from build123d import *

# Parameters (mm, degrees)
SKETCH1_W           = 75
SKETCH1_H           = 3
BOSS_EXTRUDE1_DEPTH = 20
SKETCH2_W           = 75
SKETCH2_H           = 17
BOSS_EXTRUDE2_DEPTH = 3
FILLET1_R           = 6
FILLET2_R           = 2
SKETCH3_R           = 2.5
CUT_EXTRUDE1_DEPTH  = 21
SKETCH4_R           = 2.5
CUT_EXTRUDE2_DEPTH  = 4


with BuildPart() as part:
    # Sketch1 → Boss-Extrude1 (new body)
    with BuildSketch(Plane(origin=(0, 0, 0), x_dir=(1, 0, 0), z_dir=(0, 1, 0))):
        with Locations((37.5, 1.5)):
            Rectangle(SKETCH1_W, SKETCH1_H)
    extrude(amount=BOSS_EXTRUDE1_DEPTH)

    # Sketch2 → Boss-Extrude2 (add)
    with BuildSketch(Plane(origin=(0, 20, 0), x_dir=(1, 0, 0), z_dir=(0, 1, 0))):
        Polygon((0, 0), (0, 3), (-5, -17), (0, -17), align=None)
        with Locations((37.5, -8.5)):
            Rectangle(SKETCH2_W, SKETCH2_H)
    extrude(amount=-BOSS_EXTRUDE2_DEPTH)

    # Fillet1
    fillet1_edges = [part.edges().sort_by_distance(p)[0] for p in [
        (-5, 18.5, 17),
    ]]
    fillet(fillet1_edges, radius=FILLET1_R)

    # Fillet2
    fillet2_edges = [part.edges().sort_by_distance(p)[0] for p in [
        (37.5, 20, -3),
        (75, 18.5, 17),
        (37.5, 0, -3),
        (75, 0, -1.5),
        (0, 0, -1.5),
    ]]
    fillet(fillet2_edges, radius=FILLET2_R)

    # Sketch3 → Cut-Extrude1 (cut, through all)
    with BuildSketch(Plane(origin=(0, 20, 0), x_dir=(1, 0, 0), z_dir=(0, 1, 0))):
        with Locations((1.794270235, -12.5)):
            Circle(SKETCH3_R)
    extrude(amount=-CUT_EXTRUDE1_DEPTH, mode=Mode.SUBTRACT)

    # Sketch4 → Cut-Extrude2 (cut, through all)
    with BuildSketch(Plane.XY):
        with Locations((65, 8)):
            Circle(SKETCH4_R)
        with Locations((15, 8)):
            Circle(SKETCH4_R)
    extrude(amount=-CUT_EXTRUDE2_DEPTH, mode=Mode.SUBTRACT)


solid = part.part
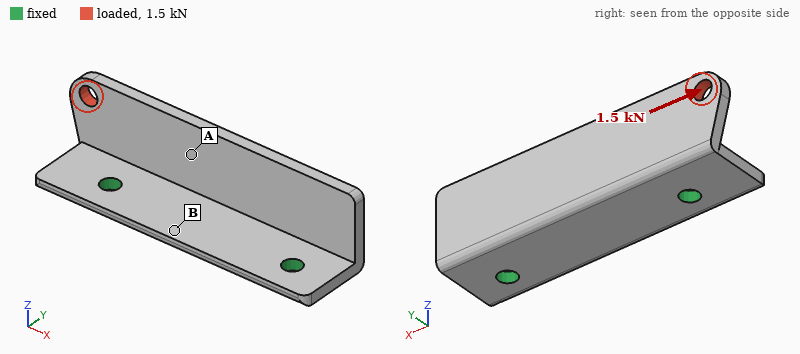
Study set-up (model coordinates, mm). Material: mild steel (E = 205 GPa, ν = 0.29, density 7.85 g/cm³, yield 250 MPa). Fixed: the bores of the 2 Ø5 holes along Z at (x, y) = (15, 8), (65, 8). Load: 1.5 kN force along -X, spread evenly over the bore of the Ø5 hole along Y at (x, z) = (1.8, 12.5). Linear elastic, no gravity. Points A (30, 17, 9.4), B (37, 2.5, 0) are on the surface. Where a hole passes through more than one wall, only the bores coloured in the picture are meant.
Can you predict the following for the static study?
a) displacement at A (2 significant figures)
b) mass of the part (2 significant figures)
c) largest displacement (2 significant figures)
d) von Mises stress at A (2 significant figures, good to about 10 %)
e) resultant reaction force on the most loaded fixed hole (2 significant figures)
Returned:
8.4 µm
64 g
37 µm
37 MPa
910 N
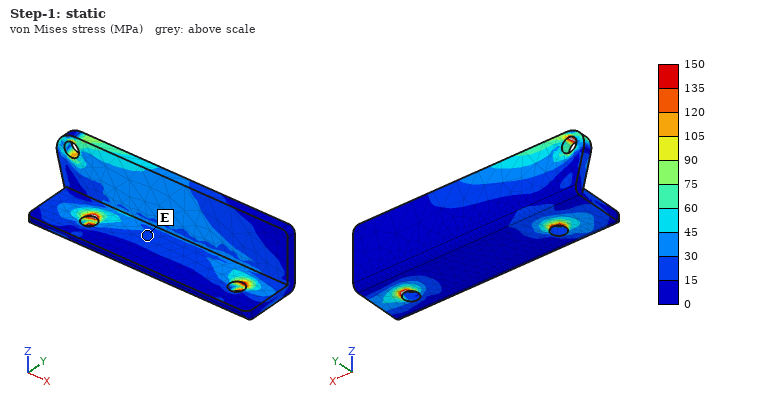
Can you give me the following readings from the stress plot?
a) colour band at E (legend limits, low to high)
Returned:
15 to 30 MPa
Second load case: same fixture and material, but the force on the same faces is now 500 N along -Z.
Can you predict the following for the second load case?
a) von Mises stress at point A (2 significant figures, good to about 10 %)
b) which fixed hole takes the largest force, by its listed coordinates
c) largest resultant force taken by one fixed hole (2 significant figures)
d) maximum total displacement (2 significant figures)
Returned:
21 MPa
(15, 8)
620 N
49 µm
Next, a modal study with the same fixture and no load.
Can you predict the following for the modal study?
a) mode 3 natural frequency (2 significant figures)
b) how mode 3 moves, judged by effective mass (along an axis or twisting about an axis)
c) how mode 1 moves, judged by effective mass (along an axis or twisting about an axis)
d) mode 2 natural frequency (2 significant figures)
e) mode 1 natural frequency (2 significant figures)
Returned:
7900 Hz
along Z
along Y
5000 Hz
3500 Hz
